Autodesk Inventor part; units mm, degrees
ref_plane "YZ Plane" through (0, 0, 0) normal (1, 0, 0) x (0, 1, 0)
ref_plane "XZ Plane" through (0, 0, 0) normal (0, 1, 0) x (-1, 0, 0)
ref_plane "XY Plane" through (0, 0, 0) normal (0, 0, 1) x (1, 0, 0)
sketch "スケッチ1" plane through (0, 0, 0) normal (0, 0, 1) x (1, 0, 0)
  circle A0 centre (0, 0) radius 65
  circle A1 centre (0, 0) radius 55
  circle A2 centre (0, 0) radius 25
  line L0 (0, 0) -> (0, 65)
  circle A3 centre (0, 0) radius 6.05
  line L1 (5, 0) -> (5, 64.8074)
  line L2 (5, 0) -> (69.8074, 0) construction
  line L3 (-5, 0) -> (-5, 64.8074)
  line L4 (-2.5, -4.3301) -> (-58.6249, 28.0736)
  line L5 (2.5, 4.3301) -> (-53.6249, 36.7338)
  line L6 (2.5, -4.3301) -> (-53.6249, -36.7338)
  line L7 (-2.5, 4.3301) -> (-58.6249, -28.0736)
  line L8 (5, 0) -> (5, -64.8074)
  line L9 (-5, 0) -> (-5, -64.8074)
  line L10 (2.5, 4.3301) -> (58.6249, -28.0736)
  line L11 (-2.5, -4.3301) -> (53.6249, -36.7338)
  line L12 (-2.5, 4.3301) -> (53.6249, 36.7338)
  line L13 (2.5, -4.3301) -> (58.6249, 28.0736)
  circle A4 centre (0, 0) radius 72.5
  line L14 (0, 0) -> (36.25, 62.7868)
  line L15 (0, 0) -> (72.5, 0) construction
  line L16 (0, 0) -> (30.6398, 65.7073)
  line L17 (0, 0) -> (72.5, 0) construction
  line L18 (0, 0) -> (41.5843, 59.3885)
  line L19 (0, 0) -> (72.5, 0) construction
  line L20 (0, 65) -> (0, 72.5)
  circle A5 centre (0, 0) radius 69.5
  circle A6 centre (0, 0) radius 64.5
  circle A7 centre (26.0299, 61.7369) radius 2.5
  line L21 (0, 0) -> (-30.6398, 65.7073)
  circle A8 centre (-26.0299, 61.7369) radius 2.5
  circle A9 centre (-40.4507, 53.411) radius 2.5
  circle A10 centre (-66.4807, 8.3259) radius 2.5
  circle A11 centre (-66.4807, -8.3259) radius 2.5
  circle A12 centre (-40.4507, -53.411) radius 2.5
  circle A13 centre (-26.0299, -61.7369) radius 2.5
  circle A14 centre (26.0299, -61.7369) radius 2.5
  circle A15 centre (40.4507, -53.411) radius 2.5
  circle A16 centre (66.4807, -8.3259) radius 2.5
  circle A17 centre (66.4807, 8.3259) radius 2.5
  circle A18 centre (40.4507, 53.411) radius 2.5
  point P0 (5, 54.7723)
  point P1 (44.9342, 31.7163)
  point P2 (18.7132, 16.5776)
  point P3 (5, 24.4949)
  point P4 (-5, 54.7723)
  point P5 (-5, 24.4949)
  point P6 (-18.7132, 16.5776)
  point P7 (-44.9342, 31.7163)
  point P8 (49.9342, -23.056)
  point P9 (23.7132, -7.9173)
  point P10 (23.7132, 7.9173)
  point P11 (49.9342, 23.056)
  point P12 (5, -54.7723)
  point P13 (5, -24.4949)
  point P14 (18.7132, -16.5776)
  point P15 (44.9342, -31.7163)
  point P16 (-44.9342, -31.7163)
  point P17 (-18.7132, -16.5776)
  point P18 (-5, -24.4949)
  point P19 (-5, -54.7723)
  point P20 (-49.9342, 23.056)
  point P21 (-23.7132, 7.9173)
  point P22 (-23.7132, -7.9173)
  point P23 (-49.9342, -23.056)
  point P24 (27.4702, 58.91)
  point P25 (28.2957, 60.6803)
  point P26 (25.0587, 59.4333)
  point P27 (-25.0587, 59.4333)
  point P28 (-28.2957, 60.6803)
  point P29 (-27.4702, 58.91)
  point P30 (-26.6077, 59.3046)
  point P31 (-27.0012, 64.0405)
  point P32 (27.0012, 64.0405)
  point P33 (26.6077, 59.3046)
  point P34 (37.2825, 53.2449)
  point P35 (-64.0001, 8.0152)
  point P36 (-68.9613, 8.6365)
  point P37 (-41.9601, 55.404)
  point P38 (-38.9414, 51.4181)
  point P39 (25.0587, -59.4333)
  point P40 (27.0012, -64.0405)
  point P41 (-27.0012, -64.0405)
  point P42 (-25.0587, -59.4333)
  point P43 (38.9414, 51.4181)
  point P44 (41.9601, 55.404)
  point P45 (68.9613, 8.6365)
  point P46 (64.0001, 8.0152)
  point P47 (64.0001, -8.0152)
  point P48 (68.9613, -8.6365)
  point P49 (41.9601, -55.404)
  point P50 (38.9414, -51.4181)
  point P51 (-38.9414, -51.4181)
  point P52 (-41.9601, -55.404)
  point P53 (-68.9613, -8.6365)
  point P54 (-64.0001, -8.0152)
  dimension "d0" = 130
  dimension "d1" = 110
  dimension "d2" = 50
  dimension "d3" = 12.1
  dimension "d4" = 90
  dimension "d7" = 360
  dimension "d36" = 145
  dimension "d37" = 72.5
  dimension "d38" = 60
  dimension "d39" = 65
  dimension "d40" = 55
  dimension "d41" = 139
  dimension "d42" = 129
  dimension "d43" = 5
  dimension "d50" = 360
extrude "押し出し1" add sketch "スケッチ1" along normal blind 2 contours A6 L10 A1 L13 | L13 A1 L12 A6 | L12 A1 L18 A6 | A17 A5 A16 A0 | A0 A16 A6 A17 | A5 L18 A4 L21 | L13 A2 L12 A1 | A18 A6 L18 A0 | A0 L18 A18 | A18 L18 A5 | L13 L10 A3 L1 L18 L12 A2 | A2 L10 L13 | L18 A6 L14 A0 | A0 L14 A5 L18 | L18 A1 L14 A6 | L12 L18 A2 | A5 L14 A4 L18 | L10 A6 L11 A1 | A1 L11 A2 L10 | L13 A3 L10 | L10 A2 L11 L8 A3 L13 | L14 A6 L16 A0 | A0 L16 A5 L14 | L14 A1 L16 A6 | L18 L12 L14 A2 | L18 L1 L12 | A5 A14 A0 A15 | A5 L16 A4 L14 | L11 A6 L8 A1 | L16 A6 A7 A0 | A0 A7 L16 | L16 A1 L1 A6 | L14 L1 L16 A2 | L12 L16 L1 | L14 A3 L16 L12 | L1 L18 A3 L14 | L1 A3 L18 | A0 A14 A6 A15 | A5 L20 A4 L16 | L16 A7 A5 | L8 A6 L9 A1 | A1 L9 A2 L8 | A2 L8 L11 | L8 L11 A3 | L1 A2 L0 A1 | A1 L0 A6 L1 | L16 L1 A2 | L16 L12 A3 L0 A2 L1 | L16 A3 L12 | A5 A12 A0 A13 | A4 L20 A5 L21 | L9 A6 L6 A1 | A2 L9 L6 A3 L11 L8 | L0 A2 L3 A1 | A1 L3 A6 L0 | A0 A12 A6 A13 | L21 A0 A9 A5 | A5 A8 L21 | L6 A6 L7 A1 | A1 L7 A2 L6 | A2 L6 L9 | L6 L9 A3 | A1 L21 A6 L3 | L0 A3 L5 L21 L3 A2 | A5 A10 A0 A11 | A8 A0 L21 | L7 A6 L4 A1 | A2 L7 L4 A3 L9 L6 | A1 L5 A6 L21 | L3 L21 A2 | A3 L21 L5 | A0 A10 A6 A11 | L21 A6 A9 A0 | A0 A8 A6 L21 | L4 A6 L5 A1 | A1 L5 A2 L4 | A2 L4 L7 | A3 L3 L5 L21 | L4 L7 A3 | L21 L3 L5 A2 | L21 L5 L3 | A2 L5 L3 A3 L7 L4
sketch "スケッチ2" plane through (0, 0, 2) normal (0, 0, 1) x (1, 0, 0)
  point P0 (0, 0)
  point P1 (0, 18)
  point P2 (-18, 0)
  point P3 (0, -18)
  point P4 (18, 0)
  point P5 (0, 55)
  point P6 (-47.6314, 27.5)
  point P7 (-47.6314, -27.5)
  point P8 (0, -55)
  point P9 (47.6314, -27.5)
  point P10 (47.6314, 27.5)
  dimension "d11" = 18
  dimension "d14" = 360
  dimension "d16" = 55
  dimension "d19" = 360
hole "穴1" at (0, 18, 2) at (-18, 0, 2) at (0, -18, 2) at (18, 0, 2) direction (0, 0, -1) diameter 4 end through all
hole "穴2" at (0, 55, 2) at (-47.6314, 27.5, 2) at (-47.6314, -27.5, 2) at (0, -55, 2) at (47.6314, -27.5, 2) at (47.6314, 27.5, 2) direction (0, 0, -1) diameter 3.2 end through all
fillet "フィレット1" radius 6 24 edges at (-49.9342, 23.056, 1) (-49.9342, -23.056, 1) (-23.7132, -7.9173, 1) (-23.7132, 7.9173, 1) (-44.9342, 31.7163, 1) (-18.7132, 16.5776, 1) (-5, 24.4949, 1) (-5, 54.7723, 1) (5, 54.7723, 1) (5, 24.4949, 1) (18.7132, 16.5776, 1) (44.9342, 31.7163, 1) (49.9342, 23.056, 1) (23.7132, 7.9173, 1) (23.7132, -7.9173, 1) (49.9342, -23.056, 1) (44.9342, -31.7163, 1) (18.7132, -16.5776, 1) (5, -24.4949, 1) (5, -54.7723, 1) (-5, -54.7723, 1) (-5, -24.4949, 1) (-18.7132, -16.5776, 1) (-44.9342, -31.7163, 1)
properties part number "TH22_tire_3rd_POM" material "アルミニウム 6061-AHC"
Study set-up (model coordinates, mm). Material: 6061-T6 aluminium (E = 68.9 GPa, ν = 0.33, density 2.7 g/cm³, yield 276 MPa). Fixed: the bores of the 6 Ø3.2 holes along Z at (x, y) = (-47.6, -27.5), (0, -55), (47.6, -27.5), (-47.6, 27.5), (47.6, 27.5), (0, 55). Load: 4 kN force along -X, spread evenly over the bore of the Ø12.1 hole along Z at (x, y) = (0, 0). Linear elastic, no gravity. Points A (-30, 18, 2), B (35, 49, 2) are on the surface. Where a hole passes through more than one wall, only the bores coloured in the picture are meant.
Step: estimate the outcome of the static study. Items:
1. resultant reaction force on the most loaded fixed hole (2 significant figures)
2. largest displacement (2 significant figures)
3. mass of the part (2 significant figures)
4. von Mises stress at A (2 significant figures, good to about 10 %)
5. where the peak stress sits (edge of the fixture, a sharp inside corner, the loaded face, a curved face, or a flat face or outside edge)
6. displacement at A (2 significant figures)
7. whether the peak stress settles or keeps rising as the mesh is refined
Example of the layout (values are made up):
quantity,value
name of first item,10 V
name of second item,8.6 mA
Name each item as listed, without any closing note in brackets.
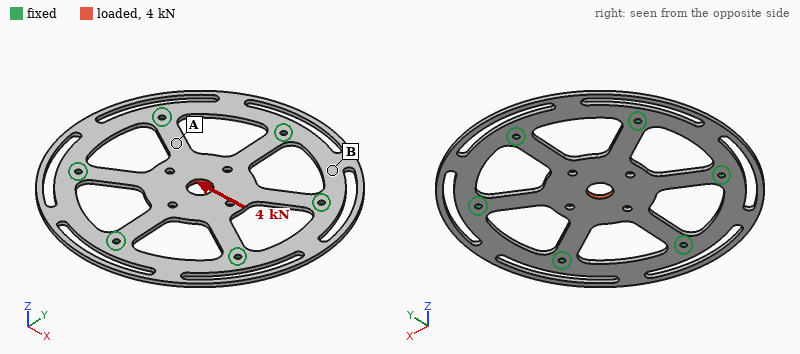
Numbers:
quantity,value
resultant reaction force on the most loaded fixed hole,1.0 kN
largest displacement,40 µm
mass of the part,49 g
von Mises stress at A,54 MPa
where the peak stress sits,edge of the fixture
displacement at A,18 µm
whether the peak stress settles or keeps rising as the mesh is refined,keeps rising
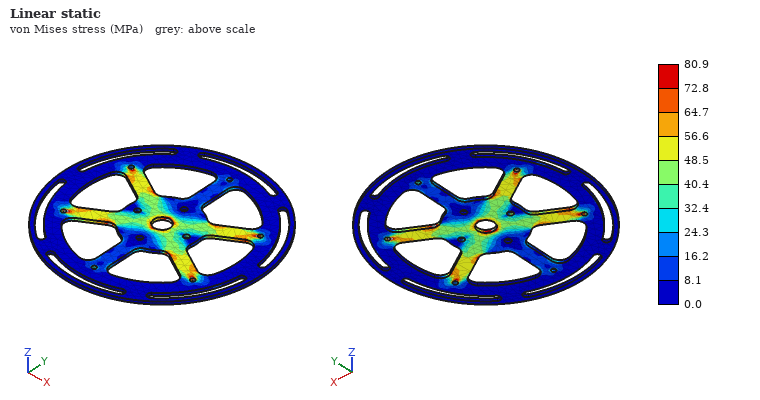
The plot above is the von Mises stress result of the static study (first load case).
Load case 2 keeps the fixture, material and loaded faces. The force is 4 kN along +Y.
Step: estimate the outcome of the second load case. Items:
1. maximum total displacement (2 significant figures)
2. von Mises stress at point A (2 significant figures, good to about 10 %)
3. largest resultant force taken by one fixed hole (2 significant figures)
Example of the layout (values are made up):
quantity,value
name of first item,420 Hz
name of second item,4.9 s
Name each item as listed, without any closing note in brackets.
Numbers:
quantity,value
maximum total displacement,42 µm
von Mises stress at point A,33 MPa
largest resultant force taken by one fixed hole,1.2 kN
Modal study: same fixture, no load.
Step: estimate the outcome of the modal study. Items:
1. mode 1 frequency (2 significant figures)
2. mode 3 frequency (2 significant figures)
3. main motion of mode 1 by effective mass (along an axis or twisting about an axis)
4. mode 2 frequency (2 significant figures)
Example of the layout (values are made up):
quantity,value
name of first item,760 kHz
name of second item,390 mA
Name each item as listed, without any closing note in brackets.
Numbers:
quantity,value
mode 1 frequency,1100 Hz
mode 3 frequency,1400 Hz
main motion of mode 1 by effective mass,along Z
mode 2 frequency,1400 Hz
